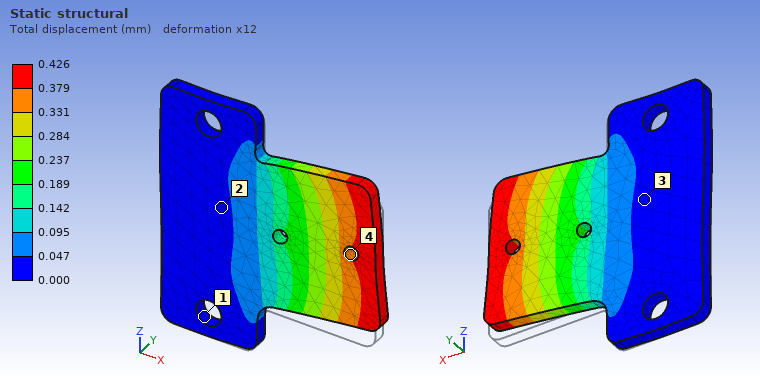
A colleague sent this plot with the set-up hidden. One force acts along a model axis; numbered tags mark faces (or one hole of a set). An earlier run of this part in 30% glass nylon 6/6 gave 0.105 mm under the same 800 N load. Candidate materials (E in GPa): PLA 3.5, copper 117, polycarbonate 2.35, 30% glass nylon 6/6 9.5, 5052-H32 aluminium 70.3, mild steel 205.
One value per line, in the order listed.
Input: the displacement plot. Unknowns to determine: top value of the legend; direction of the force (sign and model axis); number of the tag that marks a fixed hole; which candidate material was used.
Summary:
0.426 mm
+Z
1
polycarbonate
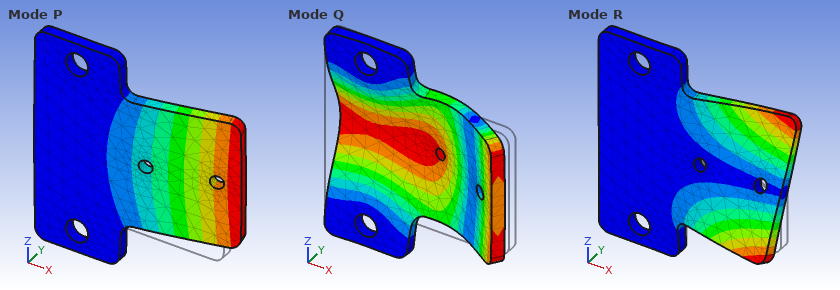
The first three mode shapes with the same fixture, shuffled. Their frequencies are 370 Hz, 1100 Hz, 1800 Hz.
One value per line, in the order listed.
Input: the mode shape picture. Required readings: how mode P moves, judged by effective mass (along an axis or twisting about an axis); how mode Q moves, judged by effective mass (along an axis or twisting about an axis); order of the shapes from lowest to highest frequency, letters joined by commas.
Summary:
along Y
along Y
P, R, Q
